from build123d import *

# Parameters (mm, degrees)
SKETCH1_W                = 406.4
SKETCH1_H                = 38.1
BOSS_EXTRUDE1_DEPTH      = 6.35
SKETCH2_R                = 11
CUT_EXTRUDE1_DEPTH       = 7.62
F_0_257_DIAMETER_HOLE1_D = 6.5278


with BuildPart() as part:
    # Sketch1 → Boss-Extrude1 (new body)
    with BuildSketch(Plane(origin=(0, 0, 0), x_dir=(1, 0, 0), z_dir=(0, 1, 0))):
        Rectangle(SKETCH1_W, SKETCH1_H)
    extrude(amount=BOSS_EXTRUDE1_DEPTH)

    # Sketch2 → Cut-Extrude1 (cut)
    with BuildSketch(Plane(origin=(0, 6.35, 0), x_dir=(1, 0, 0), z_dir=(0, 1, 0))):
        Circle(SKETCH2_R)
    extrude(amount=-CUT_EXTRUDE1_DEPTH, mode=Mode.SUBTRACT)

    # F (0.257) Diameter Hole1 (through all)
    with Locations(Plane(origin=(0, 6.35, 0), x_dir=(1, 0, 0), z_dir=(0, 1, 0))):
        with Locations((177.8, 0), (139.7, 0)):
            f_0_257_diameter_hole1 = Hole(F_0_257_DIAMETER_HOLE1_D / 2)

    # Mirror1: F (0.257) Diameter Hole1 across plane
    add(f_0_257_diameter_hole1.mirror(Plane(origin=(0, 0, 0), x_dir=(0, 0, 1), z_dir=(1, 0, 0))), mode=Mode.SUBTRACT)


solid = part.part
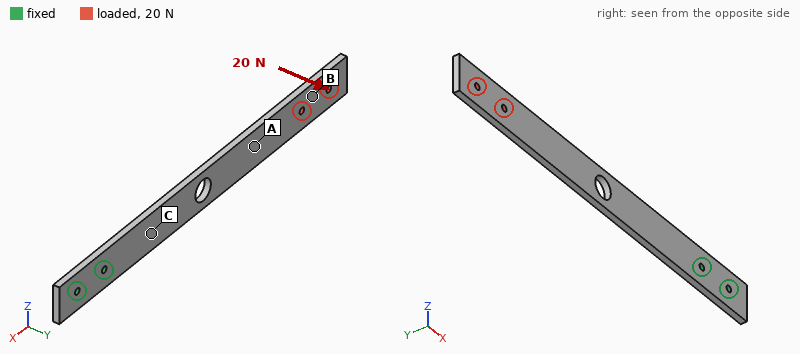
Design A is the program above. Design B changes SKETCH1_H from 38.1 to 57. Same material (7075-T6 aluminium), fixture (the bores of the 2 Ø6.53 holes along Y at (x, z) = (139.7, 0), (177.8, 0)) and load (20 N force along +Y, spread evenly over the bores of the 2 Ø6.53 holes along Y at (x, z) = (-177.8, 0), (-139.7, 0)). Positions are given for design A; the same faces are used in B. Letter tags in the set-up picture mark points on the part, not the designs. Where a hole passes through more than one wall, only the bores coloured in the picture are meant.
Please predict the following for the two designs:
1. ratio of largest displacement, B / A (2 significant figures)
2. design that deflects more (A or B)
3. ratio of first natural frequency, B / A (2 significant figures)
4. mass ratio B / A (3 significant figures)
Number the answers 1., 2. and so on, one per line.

1. 0.65
2. A
3. 1.0
4. 1.51
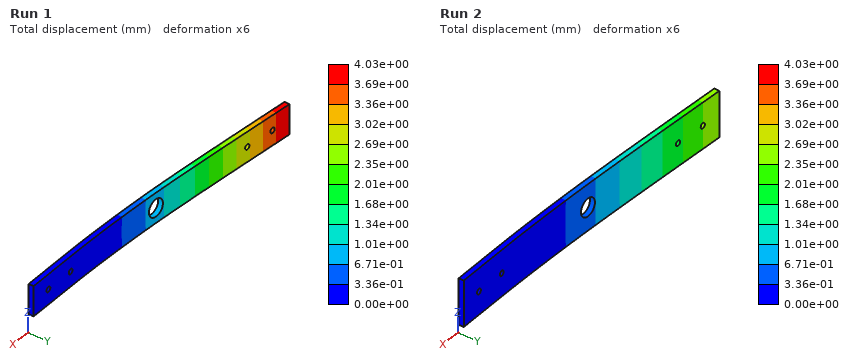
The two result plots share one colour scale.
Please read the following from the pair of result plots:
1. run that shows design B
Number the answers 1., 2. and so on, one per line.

1. Run 2
